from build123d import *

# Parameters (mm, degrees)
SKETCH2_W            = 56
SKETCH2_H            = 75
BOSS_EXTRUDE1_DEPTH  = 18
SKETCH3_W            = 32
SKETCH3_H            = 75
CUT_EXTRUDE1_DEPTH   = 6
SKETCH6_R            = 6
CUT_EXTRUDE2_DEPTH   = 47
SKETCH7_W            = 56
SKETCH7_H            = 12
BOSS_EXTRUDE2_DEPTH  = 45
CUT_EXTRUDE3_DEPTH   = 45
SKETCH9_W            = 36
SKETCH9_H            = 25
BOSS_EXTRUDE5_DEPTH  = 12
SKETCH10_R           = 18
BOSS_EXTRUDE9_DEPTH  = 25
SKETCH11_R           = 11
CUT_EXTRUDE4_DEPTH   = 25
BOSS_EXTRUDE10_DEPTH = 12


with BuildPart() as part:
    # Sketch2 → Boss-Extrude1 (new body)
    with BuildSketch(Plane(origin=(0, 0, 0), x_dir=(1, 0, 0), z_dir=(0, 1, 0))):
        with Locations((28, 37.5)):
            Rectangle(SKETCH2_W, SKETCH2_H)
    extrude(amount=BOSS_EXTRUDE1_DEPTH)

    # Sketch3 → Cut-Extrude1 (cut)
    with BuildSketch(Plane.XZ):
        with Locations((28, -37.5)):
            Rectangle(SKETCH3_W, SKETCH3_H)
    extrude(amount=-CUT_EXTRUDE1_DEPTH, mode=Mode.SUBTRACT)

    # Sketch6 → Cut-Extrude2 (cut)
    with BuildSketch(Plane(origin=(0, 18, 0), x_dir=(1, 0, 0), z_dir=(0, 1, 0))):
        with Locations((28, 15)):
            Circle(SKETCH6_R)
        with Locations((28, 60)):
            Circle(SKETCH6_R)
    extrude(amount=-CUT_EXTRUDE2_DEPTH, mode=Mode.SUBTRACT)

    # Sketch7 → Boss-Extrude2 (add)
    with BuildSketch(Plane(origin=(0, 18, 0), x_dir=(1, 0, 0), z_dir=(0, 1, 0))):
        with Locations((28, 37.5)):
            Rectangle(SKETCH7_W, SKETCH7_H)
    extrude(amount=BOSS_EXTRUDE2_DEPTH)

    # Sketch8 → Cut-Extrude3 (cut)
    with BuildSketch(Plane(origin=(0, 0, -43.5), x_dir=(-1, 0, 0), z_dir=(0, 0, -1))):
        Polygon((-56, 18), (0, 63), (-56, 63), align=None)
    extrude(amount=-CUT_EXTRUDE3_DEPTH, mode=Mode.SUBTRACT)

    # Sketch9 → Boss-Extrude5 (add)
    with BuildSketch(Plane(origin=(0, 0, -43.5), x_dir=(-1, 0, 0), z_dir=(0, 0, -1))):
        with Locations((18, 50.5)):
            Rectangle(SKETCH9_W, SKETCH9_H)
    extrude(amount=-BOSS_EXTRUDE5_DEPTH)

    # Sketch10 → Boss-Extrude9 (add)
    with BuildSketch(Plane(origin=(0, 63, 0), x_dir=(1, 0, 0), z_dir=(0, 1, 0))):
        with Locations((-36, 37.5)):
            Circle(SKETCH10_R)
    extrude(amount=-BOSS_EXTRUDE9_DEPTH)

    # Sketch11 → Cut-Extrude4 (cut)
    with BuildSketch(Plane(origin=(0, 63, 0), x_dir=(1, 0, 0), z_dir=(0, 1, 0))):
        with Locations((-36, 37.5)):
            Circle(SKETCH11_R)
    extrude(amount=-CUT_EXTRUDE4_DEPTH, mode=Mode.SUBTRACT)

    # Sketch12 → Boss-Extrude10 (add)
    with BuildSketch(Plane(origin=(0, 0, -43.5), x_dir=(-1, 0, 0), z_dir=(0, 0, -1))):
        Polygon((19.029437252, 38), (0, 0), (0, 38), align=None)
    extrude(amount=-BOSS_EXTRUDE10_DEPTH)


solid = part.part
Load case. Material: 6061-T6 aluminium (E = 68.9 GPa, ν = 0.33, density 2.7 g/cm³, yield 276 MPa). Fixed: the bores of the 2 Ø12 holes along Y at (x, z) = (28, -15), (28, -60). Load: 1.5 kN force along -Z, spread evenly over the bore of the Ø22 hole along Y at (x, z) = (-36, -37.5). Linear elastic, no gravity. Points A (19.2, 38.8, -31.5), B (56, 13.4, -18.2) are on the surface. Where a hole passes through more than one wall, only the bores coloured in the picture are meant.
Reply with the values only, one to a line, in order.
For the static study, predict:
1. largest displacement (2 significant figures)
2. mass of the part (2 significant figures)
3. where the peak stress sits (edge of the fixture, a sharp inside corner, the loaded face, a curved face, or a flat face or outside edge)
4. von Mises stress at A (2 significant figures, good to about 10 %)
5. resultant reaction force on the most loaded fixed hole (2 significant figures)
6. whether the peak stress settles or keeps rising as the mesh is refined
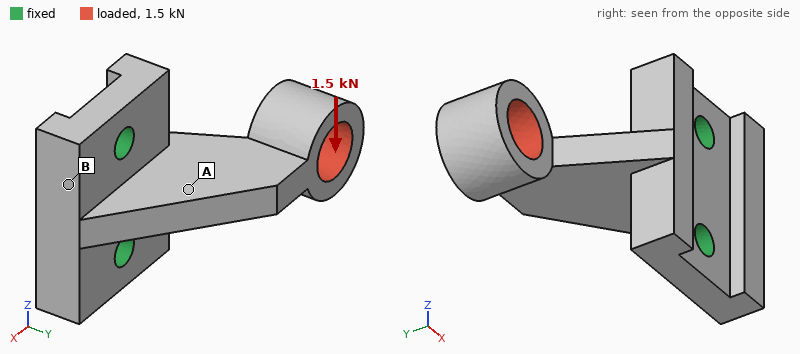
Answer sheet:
0.51 mm
270 g
a sharp inside corner
50 MPa
2.5 kN
keeps rising
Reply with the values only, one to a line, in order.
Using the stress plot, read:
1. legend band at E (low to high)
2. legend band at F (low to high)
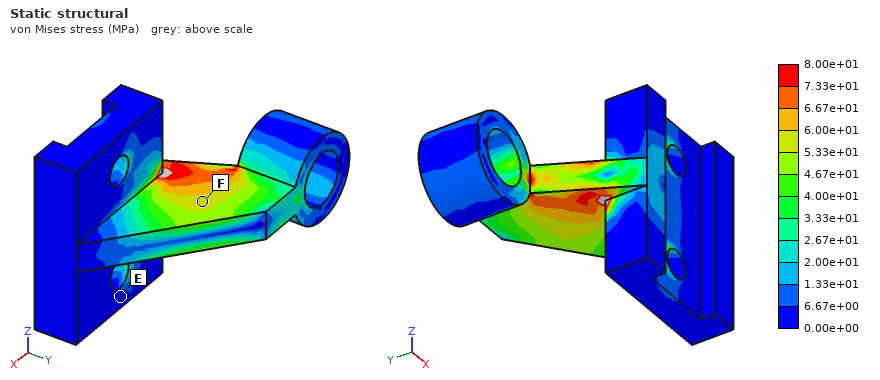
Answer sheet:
0.00e+00 to 6.67e+00 MPa
5.33e+01 to 6.00e+01 MPa
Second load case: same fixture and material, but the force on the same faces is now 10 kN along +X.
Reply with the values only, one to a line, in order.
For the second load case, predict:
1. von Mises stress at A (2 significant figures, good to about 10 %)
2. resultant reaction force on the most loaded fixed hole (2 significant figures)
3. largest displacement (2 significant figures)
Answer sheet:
58 MPa
5.1 kN
0.49 mm
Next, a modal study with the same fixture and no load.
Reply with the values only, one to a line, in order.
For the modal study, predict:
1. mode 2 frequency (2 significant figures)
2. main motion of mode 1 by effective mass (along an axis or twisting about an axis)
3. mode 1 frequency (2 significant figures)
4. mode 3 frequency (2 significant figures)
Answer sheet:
2300 Hz
along Z
1500 Hz
4000 Hz
